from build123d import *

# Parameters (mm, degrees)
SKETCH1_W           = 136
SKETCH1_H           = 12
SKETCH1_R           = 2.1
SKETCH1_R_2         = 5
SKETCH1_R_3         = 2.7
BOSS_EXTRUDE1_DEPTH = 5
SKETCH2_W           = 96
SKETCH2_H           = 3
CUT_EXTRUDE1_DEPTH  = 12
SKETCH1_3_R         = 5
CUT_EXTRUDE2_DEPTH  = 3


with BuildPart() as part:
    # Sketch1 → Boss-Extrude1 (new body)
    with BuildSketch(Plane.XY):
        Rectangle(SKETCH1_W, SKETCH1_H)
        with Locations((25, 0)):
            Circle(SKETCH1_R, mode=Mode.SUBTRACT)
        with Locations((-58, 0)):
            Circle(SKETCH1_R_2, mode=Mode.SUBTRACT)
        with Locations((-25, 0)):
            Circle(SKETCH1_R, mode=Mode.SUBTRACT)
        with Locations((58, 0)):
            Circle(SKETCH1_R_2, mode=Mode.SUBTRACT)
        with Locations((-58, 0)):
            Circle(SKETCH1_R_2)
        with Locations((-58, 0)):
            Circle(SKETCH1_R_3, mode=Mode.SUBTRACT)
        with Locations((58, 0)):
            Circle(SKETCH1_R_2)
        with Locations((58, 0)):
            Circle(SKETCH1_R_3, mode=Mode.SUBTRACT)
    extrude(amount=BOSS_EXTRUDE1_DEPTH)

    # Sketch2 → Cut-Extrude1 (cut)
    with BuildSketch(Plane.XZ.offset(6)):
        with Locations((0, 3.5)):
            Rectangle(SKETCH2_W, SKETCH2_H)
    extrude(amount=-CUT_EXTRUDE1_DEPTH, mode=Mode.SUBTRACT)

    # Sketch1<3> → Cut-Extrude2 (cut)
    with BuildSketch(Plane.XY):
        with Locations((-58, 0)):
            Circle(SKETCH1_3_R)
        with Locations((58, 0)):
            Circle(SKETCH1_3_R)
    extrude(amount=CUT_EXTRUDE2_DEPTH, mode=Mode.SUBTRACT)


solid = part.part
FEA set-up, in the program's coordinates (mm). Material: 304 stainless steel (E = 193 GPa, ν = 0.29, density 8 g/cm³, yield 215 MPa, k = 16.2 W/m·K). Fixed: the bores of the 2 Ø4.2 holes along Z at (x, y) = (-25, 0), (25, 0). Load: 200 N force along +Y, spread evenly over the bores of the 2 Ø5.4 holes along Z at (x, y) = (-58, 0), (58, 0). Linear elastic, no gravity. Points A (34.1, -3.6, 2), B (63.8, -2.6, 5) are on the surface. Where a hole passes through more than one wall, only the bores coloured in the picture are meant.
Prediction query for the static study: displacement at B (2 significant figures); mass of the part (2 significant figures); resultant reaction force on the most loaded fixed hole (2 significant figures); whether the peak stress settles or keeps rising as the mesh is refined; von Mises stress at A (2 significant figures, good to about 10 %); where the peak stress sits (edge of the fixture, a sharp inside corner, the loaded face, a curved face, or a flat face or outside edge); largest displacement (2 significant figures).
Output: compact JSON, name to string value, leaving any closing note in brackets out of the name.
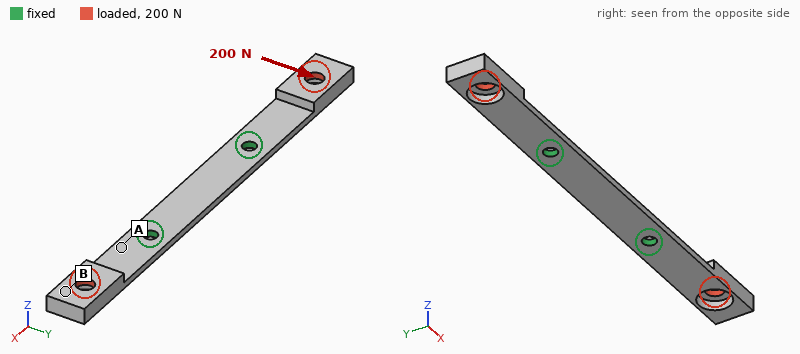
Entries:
{"displacement at B": "49 µm", "mass of the part": "33 g", "resultant reaction force on the most loaded fixed hole": "100 N", "whether the peak stress settles or keeps rising as the mesh is refined": "keeps rising", "von Mises stress at A": "49 MPa", "where the peak stress sits": "edge of the fixture", "largest displacement": "56 µm"}
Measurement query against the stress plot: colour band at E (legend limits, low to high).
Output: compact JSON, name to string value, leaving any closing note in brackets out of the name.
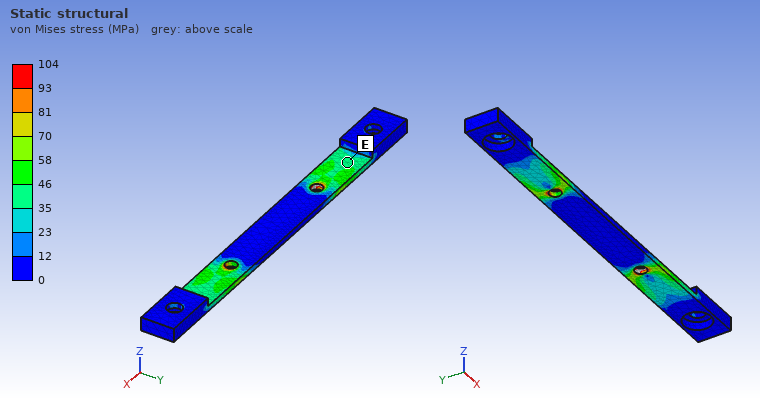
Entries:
{"colour band at E": "35 to 46 MPa"}
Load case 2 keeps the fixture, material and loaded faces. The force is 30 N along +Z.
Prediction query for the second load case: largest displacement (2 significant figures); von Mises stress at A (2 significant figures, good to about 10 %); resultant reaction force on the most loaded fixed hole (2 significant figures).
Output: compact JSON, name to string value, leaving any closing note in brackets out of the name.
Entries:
{"largest displacement": "0.14 mm", "von Mises stress at A": "44 MPa", "resultant reaction force on the most loaded fixed hole": "15 N"}
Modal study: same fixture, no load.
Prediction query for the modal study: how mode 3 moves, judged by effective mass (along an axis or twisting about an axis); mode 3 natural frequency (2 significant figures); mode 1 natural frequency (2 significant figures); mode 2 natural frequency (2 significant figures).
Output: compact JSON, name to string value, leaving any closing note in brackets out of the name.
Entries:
{"how mode 3 moves, judged by effective mass": "along Y", "mode 3 natural frequency": "3000 Hz", "mode 1 natural frequency": "680 Hz", "mode 2 natural frequency": "680 Hz"}
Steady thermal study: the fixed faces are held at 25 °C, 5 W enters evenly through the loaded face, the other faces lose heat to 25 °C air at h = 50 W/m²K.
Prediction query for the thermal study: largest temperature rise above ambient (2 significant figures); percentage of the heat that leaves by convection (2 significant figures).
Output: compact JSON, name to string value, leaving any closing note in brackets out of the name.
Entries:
{"largest temperature rise above ambient": "54 K", "percentage of the heat that leaves by convection": "84 %"}
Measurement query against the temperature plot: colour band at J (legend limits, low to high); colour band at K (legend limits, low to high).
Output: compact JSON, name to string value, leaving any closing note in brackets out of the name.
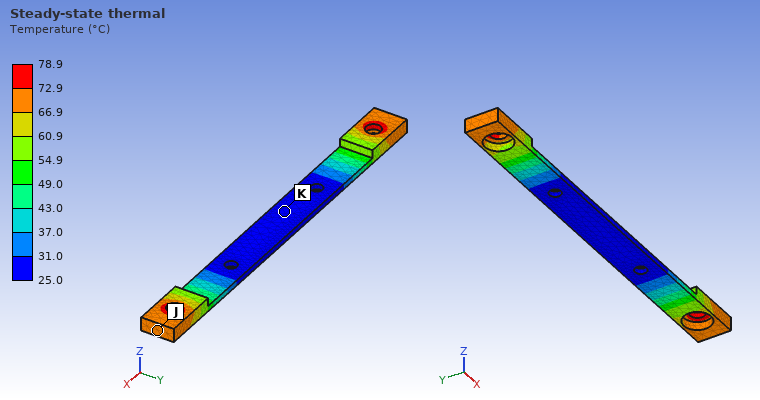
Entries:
{"colour band at J": "66.9 to 72.9 °C", "colour band at K": "25.0 to 31.0 °C"}
